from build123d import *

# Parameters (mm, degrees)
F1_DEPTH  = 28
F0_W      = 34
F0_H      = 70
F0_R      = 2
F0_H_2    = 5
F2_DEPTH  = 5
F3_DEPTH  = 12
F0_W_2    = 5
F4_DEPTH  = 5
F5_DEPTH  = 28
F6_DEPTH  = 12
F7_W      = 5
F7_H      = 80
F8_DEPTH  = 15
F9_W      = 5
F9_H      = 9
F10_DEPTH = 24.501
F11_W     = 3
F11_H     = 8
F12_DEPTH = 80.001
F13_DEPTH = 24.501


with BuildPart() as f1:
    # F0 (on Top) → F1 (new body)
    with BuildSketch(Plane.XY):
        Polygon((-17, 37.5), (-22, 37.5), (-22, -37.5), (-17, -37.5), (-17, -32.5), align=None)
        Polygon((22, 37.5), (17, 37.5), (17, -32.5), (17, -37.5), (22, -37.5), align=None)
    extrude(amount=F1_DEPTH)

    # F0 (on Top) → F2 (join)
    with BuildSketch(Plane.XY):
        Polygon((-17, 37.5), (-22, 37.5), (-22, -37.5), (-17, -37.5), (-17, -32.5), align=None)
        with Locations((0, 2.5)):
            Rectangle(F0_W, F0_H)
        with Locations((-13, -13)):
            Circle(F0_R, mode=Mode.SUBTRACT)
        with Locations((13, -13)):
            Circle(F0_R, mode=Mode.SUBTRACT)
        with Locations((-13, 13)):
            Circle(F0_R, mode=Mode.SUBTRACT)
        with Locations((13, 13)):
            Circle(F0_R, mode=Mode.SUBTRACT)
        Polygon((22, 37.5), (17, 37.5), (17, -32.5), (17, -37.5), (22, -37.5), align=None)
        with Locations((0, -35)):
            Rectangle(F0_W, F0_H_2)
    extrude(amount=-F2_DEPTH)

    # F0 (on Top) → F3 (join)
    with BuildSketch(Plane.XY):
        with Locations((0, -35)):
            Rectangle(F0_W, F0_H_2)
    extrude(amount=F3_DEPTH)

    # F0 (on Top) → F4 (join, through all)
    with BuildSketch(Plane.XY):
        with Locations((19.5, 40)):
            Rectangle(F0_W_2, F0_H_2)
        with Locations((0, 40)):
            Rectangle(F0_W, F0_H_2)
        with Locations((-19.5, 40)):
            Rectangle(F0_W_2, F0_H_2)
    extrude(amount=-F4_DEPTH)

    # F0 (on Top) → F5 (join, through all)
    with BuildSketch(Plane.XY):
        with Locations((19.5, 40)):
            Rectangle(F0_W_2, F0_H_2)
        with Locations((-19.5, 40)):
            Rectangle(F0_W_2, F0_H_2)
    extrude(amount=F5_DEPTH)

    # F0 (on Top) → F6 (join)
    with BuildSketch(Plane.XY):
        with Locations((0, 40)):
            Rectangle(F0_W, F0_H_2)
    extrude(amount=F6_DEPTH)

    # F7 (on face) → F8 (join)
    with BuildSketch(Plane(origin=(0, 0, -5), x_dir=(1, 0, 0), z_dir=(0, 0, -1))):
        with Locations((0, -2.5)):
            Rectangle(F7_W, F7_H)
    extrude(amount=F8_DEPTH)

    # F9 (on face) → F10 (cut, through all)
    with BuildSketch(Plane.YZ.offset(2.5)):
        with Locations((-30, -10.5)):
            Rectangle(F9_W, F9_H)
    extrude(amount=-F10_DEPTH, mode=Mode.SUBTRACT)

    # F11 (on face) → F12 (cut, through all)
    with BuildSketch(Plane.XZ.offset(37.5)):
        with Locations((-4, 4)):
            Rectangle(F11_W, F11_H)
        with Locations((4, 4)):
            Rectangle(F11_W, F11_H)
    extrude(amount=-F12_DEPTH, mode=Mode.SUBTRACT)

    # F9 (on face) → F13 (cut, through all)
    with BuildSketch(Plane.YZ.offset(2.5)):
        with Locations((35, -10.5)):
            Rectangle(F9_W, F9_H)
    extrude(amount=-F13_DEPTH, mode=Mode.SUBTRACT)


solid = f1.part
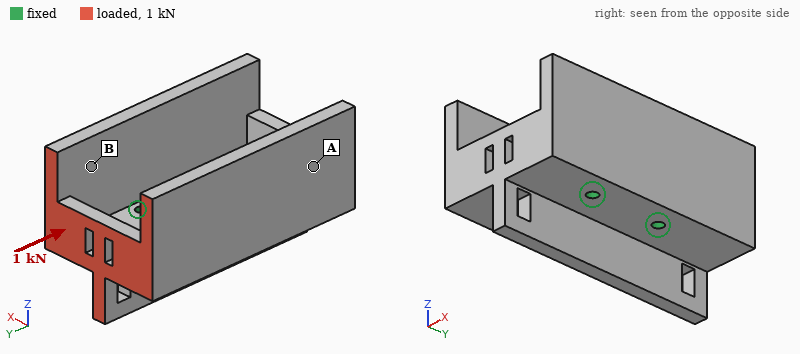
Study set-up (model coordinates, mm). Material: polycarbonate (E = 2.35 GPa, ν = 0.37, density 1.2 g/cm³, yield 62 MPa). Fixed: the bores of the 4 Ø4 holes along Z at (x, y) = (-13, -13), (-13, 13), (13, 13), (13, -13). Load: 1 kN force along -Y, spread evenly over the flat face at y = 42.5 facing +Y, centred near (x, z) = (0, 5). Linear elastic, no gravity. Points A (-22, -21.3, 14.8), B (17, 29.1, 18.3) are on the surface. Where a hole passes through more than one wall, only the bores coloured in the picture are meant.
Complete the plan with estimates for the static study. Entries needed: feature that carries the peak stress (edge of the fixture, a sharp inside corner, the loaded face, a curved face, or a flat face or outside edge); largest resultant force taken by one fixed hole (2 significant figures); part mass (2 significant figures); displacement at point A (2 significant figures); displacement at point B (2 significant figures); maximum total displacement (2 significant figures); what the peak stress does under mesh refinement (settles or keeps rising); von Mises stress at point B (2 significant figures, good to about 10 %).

edge of the fixture
360 N
59 g
0.064 mm
0.10 mm
0.28 mm
keeps rising
2.7 MPa
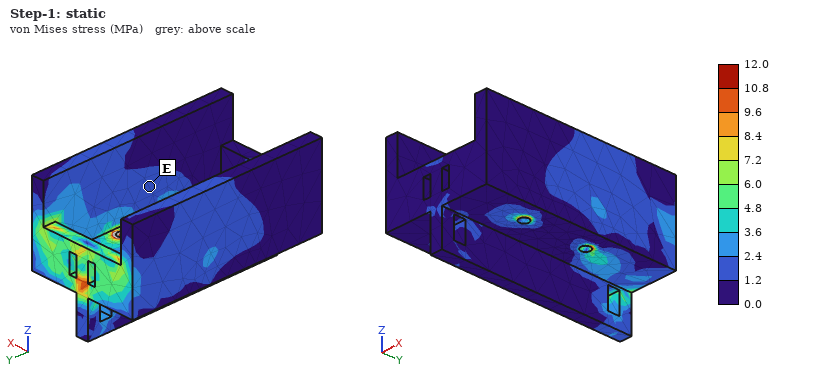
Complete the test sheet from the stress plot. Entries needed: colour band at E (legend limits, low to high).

1.2 to 2.4 MPa
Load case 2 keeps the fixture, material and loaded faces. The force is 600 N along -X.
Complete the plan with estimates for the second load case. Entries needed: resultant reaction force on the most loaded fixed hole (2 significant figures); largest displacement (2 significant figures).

590 N
0.72 mm
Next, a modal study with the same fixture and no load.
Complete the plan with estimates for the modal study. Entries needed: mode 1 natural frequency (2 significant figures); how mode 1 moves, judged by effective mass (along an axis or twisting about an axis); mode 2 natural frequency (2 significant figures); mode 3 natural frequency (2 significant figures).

1100 Hz
along X
1300 Hz
1300 Hz
